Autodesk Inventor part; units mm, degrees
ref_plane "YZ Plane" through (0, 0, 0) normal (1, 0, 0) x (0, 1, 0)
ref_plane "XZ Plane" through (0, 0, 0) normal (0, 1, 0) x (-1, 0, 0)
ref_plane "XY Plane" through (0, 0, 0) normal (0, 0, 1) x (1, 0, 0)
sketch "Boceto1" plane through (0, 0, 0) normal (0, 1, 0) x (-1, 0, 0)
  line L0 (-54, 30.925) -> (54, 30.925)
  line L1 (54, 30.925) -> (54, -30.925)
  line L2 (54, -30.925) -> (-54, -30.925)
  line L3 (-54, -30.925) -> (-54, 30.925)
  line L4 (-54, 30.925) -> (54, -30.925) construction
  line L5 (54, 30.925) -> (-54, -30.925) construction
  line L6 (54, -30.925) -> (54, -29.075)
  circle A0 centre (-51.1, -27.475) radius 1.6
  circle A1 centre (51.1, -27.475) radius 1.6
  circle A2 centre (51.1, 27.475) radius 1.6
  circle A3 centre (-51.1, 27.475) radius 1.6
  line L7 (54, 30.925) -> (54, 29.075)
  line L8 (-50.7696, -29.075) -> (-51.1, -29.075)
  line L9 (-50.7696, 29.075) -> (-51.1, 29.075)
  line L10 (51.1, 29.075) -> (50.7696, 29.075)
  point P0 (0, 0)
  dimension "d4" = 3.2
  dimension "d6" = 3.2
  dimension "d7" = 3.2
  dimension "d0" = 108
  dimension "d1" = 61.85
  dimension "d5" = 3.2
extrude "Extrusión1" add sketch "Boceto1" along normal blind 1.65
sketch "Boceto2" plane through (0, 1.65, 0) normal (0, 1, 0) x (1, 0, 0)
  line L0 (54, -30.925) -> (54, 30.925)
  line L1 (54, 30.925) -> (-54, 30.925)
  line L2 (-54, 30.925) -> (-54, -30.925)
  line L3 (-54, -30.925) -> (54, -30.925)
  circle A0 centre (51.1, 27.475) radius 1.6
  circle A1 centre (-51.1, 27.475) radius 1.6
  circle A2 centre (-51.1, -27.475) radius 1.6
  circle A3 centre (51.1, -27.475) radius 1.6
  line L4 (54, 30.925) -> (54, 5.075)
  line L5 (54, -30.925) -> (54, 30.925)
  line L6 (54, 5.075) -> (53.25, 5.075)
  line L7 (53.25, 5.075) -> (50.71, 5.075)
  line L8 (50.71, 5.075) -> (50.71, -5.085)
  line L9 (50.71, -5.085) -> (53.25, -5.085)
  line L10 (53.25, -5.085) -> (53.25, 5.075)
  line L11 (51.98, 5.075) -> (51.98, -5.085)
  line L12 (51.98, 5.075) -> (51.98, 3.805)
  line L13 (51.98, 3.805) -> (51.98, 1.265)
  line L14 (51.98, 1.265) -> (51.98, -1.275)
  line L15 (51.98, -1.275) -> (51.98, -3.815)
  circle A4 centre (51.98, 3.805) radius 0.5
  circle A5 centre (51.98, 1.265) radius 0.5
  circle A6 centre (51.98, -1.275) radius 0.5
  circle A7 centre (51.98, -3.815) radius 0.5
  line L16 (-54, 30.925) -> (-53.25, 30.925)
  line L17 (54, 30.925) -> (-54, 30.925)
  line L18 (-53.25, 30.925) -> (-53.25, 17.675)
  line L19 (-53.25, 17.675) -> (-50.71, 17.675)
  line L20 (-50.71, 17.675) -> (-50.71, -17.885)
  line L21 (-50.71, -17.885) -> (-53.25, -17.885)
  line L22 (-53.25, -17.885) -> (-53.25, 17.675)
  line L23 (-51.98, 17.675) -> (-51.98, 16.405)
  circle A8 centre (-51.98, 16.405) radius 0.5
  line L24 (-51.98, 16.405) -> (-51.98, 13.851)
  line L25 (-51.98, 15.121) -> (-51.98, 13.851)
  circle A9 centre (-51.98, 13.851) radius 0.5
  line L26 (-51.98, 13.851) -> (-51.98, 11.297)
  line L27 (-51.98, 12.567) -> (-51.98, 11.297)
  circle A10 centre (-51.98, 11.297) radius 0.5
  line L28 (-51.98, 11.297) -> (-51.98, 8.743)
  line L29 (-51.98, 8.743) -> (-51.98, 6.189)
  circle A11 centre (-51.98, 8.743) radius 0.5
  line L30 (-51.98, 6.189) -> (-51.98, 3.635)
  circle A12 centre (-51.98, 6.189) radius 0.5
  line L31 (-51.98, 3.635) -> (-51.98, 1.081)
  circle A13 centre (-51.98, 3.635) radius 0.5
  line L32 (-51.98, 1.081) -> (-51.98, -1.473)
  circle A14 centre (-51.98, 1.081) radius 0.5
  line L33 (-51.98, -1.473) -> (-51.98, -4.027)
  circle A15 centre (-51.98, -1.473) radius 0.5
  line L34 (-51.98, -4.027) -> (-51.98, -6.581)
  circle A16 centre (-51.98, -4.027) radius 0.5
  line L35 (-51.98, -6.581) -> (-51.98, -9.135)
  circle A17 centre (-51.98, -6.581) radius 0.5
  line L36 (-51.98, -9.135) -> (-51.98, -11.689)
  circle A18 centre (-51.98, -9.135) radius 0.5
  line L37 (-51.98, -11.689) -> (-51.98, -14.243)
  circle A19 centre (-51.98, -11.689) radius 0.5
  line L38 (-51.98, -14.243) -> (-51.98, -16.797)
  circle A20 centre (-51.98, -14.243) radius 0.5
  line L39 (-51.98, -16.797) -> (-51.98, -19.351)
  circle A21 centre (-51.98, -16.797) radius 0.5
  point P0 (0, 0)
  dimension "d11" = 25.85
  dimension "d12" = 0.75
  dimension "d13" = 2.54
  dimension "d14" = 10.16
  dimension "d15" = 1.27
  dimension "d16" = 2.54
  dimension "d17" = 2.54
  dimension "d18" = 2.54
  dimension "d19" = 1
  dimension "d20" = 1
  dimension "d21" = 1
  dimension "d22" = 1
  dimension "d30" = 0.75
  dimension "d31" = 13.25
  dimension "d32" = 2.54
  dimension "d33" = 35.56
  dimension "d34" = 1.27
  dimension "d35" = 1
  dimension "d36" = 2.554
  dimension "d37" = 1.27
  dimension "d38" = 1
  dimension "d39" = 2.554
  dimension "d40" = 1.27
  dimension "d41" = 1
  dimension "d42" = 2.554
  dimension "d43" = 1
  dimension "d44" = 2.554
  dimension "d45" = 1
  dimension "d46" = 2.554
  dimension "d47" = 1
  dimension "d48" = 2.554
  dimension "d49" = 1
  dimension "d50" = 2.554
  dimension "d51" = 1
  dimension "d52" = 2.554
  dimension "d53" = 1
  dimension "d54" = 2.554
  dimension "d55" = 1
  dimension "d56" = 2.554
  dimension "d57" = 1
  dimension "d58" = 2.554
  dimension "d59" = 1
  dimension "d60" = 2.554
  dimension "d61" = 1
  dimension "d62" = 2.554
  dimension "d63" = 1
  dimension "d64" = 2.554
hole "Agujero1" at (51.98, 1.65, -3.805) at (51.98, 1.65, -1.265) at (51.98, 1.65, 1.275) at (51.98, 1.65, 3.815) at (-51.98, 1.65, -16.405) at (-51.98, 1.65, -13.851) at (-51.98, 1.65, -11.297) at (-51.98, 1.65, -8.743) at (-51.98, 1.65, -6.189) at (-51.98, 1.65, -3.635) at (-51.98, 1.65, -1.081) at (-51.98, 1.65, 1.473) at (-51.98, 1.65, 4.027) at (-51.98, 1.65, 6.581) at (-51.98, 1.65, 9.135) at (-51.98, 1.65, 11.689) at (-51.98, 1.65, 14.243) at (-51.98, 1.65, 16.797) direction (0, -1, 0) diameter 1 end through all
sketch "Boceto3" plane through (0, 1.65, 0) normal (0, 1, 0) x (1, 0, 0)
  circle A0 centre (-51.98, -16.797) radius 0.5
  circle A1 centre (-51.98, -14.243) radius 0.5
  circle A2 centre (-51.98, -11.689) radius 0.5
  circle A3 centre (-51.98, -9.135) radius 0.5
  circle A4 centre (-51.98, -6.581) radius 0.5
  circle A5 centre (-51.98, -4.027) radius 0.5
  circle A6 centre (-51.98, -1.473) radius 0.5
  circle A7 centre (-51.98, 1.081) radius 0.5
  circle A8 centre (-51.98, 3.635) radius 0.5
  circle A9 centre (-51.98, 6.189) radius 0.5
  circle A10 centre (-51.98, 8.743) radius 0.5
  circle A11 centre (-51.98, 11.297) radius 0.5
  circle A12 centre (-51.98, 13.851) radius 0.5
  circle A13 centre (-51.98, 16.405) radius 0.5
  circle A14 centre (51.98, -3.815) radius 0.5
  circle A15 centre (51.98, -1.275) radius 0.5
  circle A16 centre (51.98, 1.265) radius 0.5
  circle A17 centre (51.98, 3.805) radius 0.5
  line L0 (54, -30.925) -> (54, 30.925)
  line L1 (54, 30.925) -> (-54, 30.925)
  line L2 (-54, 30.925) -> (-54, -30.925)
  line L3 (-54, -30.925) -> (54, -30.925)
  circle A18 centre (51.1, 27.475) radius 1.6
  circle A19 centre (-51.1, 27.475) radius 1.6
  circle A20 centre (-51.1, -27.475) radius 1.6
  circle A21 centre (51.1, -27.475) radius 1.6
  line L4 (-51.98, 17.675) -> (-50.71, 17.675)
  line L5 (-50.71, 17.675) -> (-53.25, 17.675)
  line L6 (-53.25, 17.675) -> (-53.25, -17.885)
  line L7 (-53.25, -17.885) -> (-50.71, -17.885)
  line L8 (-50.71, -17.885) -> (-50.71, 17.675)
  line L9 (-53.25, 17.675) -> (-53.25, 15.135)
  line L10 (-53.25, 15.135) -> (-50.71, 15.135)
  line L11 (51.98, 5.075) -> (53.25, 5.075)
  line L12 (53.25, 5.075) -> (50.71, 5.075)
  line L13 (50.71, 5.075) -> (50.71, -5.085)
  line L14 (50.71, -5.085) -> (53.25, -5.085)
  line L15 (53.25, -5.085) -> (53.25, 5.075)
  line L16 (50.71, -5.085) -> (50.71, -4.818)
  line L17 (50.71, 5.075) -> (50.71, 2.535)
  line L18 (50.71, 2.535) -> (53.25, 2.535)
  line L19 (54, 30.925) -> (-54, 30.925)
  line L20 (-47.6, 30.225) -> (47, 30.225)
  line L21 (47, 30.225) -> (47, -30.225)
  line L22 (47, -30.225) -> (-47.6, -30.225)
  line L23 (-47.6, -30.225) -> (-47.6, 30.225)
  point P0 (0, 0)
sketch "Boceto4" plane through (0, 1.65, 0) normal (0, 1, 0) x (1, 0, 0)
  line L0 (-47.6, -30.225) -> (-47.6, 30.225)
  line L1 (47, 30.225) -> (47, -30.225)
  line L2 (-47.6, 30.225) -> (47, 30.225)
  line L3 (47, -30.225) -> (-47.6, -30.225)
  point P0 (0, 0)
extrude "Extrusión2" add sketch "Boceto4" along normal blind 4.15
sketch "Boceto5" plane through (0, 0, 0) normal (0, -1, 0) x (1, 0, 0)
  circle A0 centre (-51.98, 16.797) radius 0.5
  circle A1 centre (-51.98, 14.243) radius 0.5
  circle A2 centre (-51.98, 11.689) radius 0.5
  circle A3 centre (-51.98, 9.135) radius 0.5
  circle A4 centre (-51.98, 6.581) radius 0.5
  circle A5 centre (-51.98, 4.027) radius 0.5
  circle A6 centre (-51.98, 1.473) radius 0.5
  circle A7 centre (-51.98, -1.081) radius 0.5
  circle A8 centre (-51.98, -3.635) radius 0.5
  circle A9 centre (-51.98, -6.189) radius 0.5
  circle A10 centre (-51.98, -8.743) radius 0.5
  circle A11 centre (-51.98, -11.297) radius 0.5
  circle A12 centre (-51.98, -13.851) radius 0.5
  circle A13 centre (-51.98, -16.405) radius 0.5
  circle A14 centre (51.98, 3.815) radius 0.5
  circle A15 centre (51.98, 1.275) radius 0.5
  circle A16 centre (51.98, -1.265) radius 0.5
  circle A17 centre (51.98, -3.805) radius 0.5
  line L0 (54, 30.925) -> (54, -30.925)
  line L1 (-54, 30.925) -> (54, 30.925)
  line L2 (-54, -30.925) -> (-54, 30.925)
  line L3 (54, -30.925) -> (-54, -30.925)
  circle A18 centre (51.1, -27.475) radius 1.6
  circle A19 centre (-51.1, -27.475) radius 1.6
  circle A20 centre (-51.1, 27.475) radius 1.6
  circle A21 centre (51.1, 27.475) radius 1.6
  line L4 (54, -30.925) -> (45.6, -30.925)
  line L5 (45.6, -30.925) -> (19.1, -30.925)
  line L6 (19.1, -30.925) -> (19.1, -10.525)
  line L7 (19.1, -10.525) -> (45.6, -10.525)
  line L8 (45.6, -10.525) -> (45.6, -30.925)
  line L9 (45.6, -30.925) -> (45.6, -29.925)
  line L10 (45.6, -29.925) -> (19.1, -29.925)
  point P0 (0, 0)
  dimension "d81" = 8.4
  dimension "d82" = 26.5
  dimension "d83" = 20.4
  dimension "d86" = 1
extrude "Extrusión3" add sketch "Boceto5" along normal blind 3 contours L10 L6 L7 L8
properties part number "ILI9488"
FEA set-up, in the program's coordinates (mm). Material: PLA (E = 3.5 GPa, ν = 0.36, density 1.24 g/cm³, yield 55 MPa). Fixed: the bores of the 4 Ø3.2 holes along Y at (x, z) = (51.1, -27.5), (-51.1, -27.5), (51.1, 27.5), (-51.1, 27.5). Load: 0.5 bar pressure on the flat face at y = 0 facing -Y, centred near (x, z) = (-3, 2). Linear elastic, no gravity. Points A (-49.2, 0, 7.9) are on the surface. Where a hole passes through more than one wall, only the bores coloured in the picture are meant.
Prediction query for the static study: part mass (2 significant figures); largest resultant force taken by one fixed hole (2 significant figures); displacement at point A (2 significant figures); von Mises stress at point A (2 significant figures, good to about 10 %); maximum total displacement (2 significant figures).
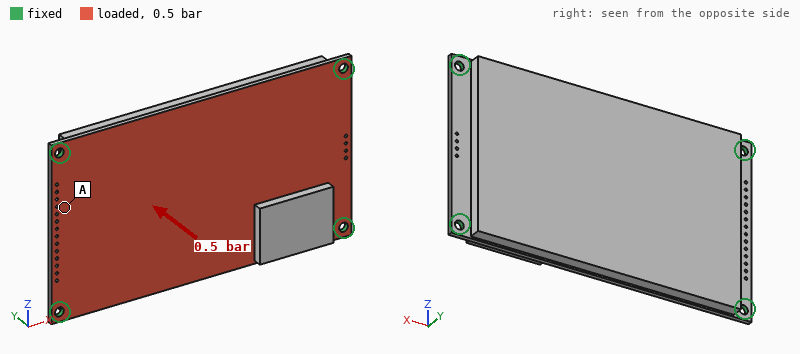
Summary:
45 g
220 N
0.14 mm
3.0 MPa
0.75 mm
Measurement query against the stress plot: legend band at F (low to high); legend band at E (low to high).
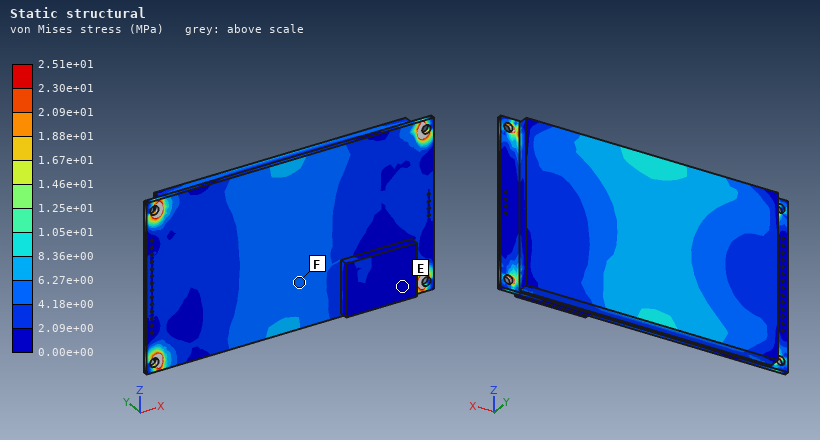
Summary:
4.18e+00 to 6.27e+00 MPa
0.00e+00 to 2.09e+00 MPa
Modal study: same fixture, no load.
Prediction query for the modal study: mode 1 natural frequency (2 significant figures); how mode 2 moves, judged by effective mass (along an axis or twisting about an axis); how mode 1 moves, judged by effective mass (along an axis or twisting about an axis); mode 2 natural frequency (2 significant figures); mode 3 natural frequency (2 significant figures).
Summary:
550 Hz
twisting about X
along Y
1100 Hz
1500 Hz
